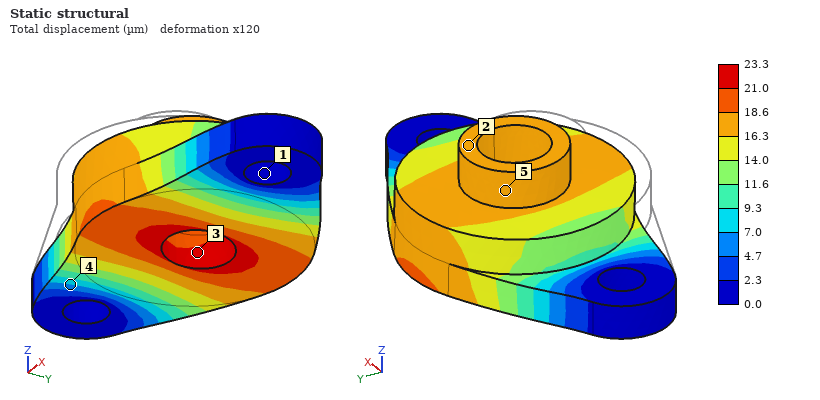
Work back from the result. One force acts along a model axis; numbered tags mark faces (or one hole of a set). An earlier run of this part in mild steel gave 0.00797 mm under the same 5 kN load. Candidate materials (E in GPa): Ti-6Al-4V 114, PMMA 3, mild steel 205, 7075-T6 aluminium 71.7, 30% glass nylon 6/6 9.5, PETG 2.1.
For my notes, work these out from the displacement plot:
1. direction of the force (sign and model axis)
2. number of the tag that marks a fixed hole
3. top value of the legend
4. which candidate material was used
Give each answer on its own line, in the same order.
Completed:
+Y
1
23.3 µm
7075-T6 aluminium
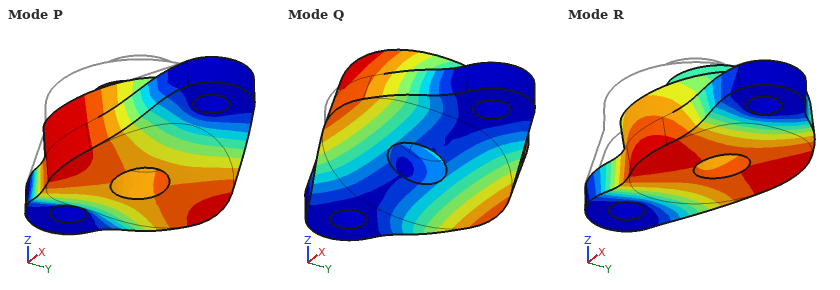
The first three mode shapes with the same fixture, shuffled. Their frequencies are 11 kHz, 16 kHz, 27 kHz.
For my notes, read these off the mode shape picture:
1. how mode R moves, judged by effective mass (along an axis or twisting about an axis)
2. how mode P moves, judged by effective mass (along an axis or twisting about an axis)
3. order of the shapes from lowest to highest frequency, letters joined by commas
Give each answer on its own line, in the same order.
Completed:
along Y
along Z
Q, P, R
